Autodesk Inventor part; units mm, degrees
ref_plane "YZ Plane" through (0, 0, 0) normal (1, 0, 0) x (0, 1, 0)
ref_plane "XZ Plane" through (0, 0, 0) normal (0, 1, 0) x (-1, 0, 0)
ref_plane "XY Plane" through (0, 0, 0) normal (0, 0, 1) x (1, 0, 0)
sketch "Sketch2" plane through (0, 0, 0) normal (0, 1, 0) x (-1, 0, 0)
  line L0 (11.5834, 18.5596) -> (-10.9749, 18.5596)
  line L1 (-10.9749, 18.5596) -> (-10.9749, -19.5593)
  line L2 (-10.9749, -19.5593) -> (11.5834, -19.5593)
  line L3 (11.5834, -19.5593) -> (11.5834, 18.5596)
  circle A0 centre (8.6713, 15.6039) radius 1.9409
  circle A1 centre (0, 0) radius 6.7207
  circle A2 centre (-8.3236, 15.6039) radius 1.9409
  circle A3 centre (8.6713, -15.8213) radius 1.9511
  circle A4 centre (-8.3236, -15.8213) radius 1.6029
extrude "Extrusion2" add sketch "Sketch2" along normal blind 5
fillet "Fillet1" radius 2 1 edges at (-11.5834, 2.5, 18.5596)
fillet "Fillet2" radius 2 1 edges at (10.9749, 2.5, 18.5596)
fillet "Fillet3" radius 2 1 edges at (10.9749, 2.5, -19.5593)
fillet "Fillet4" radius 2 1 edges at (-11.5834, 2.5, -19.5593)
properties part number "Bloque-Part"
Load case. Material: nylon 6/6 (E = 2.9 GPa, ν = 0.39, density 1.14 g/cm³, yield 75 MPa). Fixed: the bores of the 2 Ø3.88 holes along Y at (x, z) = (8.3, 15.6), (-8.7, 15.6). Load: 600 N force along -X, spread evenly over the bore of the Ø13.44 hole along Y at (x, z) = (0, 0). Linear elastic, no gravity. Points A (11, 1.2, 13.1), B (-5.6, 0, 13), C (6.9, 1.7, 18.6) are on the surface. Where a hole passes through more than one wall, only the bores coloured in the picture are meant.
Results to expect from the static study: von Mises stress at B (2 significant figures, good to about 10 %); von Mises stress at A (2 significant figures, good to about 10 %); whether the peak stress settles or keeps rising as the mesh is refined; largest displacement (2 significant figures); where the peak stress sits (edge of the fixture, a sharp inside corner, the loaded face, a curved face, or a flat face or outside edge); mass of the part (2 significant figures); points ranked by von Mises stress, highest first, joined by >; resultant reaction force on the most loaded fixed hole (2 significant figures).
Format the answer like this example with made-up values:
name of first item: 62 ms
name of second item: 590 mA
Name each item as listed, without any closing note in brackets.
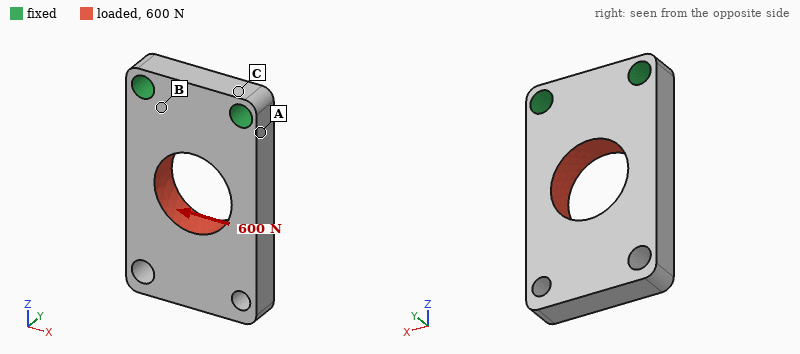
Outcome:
von Mises stress at B: 11 MPa
von Mises stress at A: 23 MPa
whether the peak stress settles or keeps rising as the mesh is refined: keeps rising
largest displacement: 0.49 mm
where the peak stress sits: edge of the fixture
mass of the part: 3.8 g
points ranked by von Mises stress, highest first, joined by >: A > B > C
resultant reaction force on the most loaded fixed hole: 570 N
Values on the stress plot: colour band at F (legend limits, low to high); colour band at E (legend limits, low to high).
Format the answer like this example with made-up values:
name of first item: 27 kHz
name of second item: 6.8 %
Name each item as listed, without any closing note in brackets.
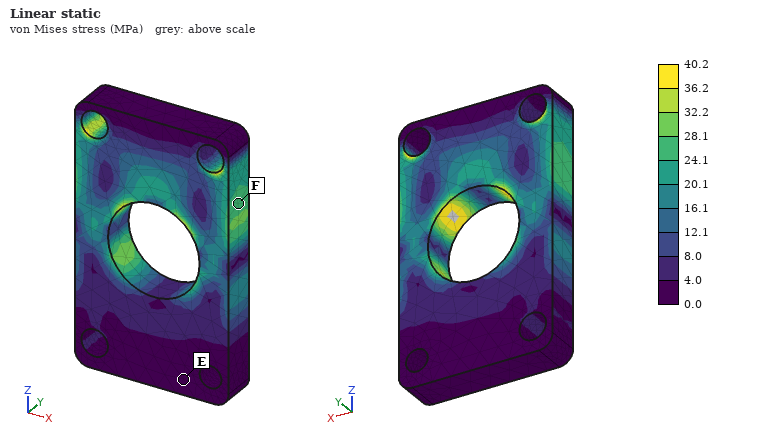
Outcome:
colour band at F: 24.1 to 28.1 MPa
colour band at E: 0.0 to 4.0 MPa
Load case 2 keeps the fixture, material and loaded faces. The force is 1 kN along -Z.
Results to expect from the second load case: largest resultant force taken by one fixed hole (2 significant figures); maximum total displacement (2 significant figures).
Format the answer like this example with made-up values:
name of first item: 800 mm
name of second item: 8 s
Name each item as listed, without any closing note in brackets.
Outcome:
largest resultant force taken by one fixed hole: 520 N
maximum total displacement: 0.11 mm
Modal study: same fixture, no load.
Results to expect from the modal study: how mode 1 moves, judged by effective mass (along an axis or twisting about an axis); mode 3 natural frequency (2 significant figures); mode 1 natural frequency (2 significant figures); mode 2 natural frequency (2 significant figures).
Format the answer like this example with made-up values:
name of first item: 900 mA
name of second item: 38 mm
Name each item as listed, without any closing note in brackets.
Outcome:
how mode 1 moves, judged by effective mass: along Y
mode 3 natural frequency: 2900 Hz
mode 1 natural frequency: 940 Hz
mode 2 natural frequency: 2900 Hz
